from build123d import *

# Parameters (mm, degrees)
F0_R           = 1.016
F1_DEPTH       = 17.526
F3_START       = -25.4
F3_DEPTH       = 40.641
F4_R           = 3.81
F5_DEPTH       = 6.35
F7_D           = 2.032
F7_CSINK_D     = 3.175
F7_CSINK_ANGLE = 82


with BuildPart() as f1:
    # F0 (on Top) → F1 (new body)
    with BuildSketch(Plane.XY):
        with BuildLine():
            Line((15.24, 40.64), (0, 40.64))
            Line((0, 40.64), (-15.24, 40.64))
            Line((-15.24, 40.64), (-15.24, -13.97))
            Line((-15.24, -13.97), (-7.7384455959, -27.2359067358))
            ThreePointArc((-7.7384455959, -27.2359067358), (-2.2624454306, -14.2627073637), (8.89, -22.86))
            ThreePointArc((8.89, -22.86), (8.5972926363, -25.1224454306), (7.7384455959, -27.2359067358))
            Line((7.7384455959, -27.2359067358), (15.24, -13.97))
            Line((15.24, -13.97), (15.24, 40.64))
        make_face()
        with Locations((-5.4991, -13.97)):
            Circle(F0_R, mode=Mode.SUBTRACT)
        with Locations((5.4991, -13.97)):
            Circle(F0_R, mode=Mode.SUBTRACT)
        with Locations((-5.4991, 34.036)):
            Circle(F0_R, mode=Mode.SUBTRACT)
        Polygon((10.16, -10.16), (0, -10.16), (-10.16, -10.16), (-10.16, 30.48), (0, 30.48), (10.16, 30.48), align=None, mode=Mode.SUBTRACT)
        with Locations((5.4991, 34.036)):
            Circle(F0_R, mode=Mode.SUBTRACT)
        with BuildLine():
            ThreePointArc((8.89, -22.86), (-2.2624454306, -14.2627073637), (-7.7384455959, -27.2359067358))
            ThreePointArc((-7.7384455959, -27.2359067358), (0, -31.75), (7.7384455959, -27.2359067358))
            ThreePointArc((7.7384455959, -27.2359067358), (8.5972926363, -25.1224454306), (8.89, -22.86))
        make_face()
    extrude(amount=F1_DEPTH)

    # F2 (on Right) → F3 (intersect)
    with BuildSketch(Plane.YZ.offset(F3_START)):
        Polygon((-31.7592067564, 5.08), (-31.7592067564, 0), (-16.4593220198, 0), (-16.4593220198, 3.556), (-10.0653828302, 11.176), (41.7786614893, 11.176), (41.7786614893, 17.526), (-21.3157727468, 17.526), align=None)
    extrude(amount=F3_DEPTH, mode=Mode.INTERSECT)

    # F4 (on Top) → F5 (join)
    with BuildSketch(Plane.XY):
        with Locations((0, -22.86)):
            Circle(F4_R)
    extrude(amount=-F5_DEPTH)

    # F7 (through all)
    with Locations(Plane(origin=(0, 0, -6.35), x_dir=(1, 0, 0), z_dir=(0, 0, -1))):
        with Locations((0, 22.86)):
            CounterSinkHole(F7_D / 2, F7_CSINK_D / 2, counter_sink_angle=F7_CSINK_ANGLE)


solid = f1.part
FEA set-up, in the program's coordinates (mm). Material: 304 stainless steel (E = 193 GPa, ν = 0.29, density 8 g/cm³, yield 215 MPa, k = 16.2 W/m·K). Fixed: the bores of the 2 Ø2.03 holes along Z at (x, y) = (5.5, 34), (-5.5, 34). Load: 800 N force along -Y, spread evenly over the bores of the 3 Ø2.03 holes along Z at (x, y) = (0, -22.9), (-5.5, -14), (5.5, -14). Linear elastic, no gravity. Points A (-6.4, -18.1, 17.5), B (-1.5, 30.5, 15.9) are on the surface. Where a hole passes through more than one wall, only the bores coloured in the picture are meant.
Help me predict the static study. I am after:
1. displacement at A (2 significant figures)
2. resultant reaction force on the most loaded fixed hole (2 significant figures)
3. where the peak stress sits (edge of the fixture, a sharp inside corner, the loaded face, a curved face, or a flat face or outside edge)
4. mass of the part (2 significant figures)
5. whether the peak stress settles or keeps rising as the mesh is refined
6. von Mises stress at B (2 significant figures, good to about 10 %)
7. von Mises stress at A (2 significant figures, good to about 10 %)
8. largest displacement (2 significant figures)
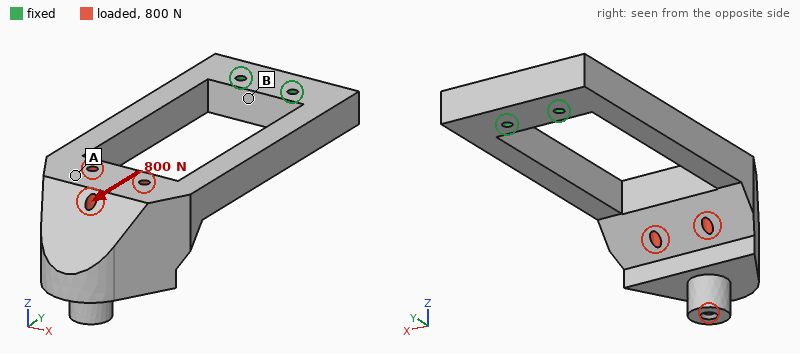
0.17 mm
450 N
a sharp inside corner
86 g
keeps rising
14 MPa
7.8 MPa
0.26 mm
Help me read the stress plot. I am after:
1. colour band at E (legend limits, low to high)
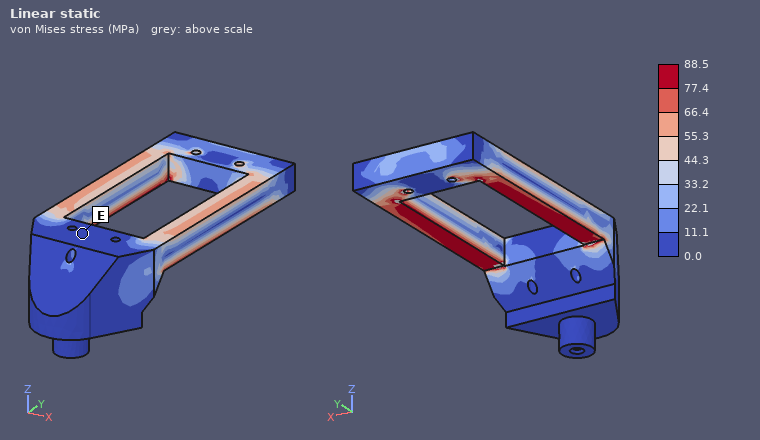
0.0 to 11.1 MPa
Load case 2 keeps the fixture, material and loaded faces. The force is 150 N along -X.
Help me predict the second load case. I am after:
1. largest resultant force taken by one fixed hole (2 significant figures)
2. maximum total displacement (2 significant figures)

560 N
80 µm
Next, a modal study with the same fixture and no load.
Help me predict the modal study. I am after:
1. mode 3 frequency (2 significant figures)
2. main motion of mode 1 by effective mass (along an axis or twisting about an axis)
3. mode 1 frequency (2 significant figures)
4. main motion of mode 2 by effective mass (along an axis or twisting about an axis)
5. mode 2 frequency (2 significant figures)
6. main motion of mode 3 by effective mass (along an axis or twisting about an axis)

2300 Hz
along Z
560 Hz
along X
1000 Hz
twisting about Y
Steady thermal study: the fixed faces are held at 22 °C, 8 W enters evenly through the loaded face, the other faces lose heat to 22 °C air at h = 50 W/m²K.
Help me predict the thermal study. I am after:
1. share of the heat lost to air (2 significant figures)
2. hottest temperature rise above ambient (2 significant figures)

94 %
61 K
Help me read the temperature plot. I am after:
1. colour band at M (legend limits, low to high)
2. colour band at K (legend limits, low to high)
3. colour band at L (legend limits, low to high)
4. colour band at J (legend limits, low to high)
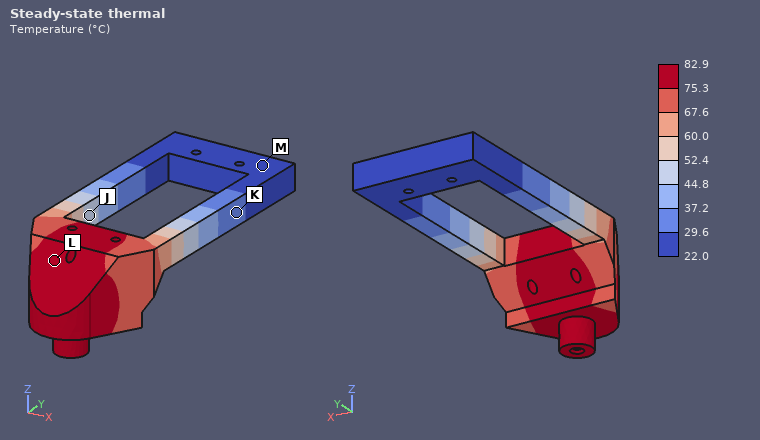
22.0 to 29.6 °C
29.6 to 37.2 °C
75.3 to 82.9 °C
44.8 to 52.4 °C
